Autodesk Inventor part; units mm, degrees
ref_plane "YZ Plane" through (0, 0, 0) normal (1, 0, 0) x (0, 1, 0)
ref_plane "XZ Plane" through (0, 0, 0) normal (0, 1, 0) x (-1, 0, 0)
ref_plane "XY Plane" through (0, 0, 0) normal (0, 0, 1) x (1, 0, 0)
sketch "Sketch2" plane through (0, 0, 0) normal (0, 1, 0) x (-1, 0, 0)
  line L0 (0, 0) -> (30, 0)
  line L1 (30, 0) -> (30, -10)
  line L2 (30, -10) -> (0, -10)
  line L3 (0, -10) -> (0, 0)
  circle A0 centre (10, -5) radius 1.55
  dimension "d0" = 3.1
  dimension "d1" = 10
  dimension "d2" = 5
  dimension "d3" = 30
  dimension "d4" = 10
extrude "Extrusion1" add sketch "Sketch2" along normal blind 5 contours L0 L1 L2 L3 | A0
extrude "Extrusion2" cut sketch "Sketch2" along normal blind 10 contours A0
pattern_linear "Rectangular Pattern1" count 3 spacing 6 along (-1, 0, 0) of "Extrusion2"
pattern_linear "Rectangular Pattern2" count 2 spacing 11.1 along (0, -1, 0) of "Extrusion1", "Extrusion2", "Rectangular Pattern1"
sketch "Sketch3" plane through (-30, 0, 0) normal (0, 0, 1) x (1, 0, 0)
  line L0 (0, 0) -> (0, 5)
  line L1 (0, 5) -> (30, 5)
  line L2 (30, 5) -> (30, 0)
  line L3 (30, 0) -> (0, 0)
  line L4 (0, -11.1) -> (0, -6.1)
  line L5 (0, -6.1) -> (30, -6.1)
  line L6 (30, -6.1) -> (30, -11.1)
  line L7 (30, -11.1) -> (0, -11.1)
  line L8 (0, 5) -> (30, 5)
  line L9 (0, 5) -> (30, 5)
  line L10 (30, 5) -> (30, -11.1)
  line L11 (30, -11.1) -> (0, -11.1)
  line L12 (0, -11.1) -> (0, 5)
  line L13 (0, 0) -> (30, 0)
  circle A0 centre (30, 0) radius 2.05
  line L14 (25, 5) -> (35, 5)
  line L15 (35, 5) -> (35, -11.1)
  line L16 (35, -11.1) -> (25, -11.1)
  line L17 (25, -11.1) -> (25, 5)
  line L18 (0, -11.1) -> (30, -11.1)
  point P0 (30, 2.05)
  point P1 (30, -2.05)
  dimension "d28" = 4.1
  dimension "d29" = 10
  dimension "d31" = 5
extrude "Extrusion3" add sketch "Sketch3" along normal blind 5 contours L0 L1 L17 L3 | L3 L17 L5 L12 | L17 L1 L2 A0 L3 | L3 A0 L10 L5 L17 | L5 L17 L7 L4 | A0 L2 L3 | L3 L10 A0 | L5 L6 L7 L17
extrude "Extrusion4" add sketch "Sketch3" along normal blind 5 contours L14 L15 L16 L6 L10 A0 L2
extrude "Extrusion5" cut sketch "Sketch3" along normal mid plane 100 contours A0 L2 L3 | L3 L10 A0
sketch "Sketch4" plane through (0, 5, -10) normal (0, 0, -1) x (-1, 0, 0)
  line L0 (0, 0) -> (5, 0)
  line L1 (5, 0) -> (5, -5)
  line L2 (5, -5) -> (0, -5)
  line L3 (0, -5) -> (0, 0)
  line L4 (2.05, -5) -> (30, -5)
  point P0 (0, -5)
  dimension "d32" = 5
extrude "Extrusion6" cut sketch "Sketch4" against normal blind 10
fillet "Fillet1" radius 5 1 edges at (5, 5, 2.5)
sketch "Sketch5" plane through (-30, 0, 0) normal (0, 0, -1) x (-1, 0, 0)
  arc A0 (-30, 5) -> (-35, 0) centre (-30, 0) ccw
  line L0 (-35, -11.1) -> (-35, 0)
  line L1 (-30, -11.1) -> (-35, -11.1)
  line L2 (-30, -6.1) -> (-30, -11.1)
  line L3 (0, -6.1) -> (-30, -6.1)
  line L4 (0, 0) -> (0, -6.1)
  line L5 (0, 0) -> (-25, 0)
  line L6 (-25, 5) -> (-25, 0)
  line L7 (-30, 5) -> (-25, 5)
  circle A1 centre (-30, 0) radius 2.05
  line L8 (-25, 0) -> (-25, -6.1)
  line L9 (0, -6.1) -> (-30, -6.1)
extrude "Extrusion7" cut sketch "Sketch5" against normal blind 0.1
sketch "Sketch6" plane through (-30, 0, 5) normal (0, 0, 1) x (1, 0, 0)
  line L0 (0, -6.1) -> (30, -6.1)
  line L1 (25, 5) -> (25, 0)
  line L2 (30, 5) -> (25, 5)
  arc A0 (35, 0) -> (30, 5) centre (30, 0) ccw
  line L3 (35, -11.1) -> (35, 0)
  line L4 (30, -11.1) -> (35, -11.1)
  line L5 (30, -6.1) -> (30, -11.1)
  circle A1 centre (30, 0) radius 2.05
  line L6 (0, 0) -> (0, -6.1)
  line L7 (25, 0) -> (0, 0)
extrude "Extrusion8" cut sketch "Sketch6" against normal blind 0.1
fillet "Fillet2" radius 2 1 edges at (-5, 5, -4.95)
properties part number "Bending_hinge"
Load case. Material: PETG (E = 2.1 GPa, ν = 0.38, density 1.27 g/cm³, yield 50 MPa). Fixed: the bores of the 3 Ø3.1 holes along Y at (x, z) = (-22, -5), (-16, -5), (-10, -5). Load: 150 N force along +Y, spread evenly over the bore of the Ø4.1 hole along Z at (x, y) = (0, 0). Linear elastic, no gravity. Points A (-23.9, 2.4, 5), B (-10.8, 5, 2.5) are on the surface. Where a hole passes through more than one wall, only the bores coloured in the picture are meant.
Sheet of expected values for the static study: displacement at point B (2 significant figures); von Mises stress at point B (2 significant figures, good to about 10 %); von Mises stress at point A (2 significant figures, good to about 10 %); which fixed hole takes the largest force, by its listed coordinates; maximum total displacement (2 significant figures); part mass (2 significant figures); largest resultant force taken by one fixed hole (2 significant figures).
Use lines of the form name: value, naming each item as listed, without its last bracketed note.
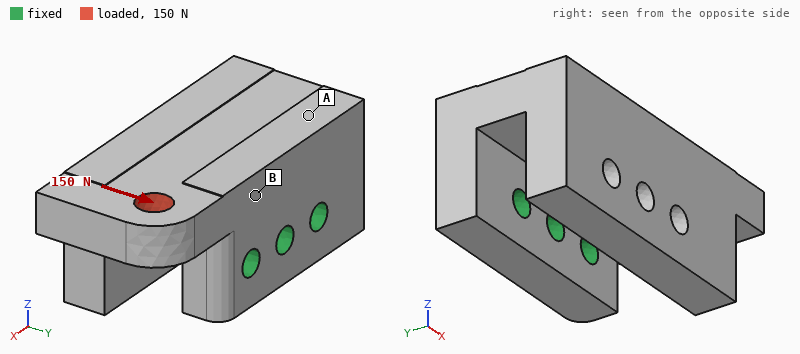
displacement at point B: 0.091 mm
von Mises stress at point B: 7.7 MPa
von Mises stress at point A: 3.2 MPa
which fixed hole takes the largest force, by its listed coordinates: (-10, -5)
maximum total displacement: 0.39 mm
part mass: 6.6 g
largest resultant force taken by one fixed hole: 190 N
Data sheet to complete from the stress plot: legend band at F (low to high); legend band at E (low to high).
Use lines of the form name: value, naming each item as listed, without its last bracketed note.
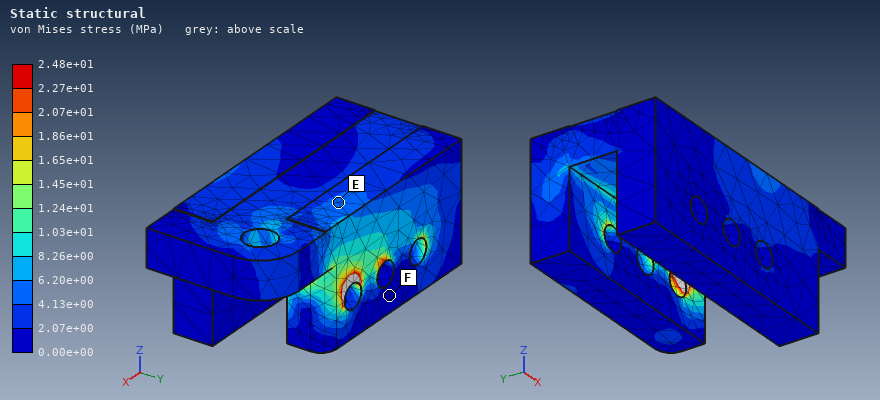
legend band at F: 0.00e+00 to 2.07e+00 MPa
legend band at E: 4.13e+00 to 6.20e+00 MPa
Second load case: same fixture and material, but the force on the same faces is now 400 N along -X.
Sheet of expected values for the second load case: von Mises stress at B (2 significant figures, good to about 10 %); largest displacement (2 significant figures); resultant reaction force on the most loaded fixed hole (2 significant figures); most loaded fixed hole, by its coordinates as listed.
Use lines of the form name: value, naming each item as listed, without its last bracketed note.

von Mises stress at B: 7.1 MPa
largest displacement: 0.15 mm
resultant reaction force on the most loaded fixed hole: 260 N
most loaded fixed hole, by its coordinates as listed: (-10, -5)
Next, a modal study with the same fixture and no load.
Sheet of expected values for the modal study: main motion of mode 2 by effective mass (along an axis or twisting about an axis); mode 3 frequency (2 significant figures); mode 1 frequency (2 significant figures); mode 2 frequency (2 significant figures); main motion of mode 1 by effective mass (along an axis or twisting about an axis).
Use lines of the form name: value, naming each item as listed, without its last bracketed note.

main motion of mode 2 by effective mass: along X
mode 3 frequency: 3400 Hz
mode 1 frequency: 1700 Hz
mode 2 frequency: 2300 Hz
main motion of mode 1 by effective mass: along Z
